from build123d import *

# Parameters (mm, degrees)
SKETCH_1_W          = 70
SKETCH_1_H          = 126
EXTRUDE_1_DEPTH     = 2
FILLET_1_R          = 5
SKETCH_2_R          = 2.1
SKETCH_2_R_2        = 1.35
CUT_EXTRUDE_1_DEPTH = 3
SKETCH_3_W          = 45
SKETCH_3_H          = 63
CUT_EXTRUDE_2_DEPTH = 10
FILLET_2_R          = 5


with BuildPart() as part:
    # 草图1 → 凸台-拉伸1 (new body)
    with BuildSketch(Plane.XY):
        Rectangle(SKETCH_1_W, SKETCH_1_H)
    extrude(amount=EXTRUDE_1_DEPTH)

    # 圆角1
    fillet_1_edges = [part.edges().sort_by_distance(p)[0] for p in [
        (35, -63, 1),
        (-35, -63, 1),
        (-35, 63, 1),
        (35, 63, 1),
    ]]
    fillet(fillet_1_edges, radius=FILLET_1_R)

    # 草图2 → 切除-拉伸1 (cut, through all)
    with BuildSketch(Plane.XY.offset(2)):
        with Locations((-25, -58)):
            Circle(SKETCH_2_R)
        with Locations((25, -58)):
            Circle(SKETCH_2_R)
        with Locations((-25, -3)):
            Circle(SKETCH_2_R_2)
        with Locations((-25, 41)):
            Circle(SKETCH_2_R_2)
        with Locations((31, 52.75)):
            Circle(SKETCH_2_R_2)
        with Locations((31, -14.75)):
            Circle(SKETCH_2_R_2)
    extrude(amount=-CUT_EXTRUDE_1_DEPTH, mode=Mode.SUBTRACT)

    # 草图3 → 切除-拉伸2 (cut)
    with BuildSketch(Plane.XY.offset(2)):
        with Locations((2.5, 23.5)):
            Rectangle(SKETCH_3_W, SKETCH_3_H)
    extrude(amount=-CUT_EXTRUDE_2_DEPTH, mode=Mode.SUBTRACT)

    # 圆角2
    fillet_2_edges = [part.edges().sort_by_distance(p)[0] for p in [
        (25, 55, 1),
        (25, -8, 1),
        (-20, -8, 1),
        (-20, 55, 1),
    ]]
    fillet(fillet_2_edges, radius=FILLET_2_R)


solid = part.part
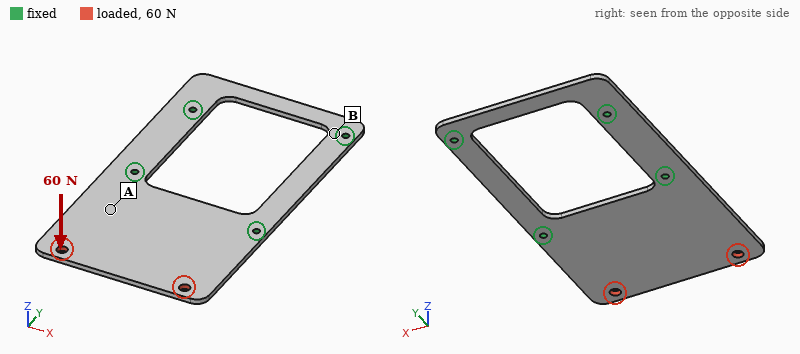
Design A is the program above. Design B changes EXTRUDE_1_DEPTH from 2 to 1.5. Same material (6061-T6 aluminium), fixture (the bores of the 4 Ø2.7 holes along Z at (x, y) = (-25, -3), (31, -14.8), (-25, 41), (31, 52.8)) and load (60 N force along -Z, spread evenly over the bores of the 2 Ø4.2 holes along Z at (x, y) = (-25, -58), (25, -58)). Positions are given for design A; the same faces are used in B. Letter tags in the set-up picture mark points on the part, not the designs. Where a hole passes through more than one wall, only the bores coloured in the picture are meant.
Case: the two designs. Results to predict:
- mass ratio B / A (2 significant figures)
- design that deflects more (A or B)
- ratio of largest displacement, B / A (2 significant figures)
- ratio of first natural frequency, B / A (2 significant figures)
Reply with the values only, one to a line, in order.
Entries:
0.75
B
2.3
0.76
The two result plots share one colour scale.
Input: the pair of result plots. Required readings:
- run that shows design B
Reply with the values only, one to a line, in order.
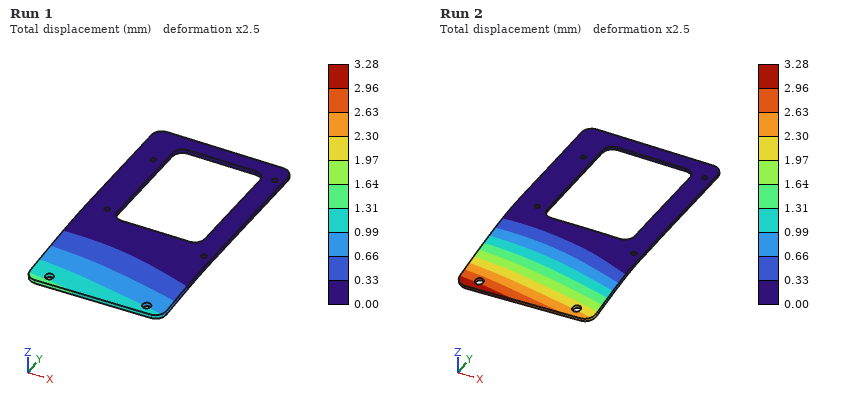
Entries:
Run 2
